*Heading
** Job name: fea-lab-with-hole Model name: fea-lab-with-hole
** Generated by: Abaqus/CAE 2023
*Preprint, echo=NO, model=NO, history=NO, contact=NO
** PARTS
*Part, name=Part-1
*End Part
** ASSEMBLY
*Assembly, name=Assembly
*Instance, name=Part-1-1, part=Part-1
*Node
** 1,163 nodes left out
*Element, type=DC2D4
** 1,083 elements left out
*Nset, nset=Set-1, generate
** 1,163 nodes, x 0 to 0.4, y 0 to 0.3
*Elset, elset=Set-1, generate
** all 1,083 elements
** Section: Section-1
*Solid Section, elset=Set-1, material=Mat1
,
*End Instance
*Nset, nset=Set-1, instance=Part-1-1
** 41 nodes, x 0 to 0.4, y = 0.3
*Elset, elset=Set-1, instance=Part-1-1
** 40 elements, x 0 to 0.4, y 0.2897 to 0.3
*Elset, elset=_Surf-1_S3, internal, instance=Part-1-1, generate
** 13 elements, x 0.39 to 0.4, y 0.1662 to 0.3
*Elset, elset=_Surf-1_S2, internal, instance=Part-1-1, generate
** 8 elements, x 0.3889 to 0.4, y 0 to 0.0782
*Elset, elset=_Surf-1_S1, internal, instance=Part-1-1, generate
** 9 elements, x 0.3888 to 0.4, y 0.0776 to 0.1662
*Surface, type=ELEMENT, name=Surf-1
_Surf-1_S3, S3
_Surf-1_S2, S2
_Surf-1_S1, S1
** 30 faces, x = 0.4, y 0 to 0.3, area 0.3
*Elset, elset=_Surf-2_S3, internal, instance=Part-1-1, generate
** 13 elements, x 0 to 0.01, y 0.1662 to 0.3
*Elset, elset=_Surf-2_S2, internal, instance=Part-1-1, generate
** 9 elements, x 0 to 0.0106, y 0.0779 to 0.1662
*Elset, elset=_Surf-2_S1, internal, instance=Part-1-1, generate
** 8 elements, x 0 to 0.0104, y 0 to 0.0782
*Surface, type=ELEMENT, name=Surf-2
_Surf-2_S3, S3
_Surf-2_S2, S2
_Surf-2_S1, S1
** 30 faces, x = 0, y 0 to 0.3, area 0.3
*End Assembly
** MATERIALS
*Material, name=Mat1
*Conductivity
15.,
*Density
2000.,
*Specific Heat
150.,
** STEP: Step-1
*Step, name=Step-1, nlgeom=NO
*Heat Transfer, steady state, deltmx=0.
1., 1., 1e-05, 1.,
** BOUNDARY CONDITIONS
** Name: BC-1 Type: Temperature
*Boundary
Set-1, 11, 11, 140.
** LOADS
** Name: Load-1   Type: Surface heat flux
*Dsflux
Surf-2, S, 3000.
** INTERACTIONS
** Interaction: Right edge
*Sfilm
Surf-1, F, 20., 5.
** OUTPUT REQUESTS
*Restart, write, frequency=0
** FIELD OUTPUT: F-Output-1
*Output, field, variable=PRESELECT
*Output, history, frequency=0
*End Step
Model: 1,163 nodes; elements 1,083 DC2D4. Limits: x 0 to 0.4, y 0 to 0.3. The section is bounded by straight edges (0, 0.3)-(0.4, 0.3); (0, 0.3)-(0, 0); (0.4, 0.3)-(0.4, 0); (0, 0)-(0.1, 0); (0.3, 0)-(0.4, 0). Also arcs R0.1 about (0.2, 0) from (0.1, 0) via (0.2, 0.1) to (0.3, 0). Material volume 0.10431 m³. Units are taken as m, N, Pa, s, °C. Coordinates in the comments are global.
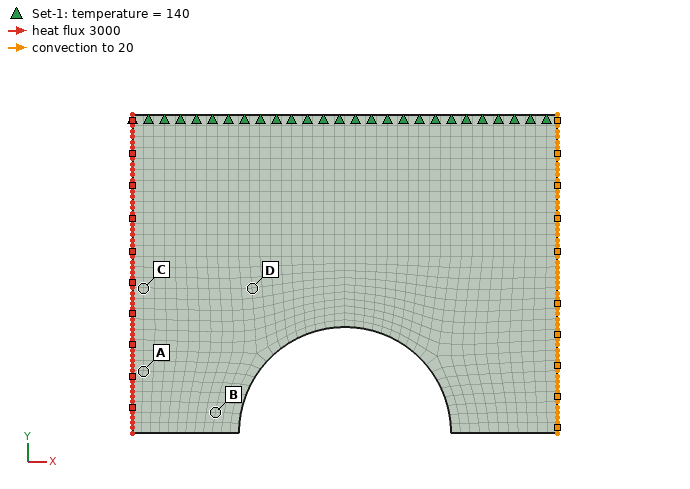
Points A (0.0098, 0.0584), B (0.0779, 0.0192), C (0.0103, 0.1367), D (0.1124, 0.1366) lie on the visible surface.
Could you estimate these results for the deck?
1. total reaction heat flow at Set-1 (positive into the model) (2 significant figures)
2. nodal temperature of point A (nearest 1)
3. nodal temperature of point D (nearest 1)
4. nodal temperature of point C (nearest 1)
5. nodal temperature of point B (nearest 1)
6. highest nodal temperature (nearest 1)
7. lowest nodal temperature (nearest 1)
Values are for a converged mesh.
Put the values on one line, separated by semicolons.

-720 W; 188 °C; 164 °C; 180 °C; 181 °C; 192 °C; 137 °C
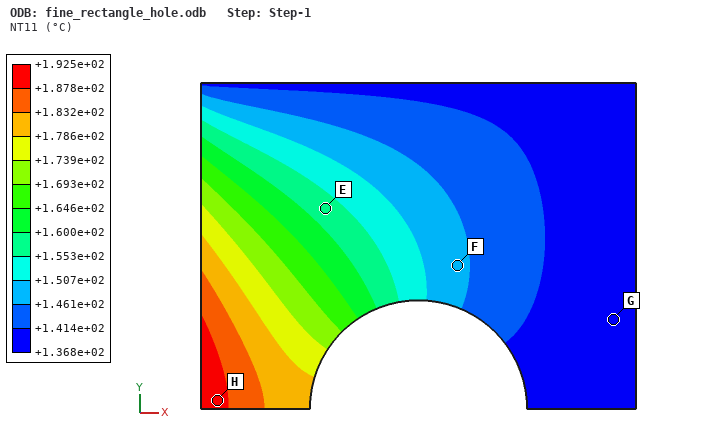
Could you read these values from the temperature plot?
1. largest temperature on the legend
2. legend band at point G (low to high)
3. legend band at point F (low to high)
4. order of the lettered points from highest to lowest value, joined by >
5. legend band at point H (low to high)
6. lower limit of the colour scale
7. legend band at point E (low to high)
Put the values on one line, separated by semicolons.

+1.925e+02 °C; +1.368e+02 to +1.414e+02 °C; +1.461e+02 to +1.507e+02 °C; H > E > F > G; +1.878e+02 to +1.925e+02 °C; +1.368e+02 °C; +1.553e+02 to +1.600e+02 °C
